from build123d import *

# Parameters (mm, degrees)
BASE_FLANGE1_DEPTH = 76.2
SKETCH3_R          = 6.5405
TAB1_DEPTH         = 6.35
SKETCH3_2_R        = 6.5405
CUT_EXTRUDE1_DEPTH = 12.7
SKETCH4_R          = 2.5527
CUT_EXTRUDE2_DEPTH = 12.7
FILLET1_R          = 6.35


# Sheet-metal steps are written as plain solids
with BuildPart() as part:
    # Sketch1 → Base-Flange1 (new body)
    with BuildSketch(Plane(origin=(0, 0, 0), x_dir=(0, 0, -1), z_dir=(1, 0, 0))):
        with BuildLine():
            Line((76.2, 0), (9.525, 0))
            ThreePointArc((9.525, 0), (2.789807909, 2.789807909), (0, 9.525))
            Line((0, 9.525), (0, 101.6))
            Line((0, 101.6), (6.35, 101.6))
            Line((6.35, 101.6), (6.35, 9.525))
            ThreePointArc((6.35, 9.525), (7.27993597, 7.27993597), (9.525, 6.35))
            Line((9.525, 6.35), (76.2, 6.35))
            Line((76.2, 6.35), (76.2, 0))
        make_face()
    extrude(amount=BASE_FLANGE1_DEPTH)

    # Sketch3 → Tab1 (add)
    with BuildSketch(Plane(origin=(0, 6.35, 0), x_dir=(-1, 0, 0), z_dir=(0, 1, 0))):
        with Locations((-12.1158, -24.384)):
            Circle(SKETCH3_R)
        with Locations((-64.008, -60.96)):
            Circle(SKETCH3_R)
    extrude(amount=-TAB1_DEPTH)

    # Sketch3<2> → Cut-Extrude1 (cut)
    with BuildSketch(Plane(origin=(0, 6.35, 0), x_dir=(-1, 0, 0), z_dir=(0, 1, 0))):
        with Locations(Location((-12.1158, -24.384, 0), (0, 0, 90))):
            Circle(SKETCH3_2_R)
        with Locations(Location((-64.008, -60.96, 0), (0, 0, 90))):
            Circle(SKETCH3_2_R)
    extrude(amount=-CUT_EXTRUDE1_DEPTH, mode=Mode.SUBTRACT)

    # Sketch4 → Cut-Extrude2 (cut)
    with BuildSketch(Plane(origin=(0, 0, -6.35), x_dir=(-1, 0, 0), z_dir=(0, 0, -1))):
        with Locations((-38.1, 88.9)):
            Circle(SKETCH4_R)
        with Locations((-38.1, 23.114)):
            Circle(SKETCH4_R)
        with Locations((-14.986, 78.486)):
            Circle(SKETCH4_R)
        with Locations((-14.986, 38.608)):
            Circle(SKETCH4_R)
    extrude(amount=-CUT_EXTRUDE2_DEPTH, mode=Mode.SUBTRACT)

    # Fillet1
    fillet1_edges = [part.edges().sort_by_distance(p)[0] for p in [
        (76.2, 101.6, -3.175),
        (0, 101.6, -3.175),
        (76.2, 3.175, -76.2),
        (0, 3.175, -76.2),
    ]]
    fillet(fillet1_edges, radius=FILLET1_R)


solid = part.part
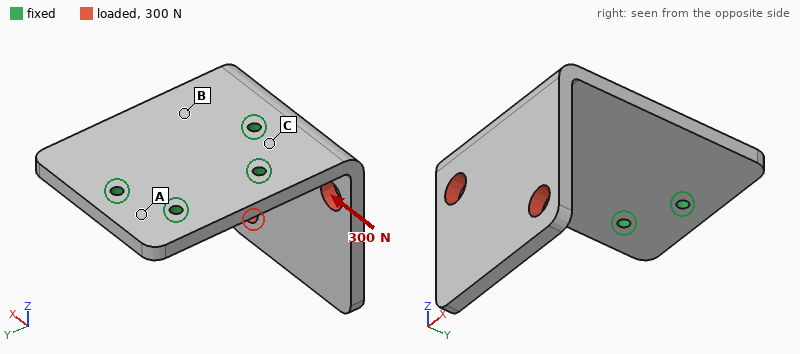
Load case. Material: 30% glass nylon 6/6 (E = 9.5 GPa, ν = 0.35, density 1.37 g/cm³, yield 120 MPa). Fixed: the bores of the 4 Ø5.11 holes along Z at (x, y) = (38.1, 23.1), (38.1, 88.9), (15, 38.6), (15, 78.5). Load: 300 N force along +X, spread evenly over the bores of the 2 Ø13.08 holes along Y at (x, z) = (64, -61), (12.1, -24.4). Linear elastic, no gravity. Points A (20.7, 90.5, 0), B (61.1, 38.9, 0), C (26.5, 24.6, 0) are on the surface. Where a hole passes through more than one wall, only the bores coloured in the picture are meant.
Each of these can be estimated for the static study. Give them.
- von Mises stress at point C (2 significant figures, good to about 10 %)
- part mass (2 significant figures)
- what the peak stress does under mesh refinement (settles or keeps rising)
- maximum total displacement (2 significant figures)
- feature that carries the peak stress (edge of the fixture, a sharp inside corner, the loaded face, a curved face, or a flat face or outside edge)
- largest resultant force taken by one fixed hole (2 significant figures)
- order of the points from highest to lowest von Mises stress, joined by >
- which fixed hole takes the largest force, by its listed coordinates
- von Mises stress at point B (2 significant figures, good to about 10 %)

11 MPa
110 g
keeps rising
0.76 mm
edge of the fixture
380 N
C > B > A
(38.1, 23.1)
6.6 MPa
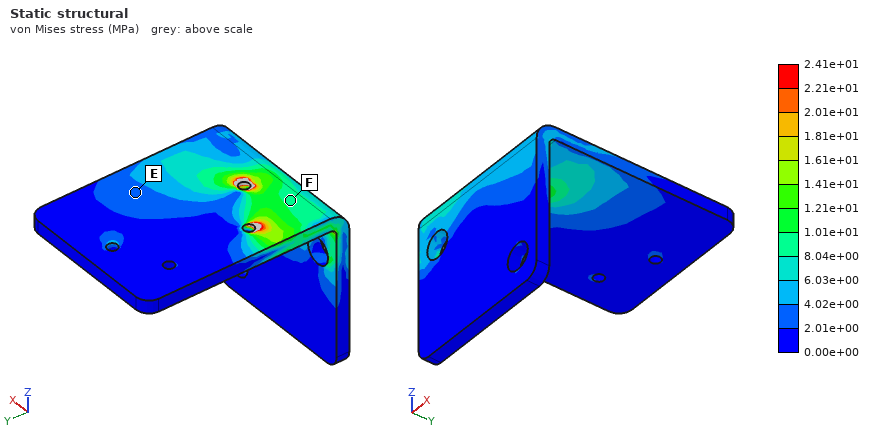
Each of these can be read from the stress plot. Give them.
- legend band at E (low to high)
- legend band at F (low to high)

2.01e+00 to 4.02e+00 MPa
8.04e+00 to 1.01e+01 MPa
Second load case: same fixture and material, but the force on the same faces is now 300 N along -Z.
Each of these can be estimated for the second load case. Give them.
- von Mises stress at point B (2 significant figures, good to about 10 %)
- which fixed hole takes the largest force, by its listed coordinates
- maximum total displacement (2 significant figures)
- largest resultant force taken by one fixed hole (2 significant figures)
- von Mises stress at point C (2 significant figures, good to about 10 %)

2.8 MPa
(38.1, 23.1)
0.43 mm
350 N
6.7 MPa
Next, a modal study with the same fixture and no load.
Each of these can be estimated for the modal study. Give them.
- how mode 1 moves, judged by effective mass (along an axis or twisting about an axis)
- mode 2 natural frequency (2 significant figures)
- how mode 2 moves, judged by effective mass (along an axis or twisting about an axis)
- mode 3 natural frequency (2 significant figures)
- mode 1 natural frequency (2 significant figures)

along Y
550 Hz
along X
1100 Hz
350 Hz
